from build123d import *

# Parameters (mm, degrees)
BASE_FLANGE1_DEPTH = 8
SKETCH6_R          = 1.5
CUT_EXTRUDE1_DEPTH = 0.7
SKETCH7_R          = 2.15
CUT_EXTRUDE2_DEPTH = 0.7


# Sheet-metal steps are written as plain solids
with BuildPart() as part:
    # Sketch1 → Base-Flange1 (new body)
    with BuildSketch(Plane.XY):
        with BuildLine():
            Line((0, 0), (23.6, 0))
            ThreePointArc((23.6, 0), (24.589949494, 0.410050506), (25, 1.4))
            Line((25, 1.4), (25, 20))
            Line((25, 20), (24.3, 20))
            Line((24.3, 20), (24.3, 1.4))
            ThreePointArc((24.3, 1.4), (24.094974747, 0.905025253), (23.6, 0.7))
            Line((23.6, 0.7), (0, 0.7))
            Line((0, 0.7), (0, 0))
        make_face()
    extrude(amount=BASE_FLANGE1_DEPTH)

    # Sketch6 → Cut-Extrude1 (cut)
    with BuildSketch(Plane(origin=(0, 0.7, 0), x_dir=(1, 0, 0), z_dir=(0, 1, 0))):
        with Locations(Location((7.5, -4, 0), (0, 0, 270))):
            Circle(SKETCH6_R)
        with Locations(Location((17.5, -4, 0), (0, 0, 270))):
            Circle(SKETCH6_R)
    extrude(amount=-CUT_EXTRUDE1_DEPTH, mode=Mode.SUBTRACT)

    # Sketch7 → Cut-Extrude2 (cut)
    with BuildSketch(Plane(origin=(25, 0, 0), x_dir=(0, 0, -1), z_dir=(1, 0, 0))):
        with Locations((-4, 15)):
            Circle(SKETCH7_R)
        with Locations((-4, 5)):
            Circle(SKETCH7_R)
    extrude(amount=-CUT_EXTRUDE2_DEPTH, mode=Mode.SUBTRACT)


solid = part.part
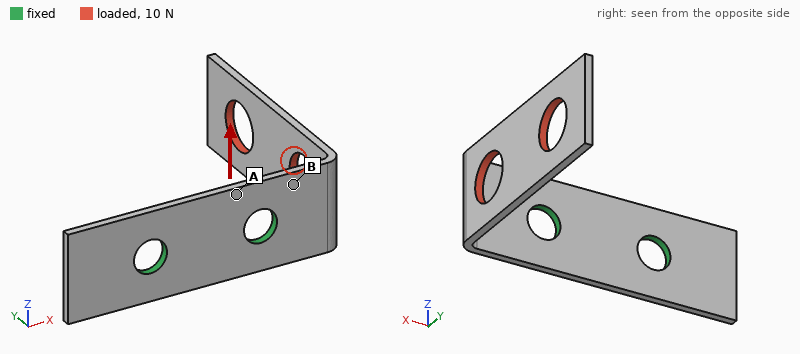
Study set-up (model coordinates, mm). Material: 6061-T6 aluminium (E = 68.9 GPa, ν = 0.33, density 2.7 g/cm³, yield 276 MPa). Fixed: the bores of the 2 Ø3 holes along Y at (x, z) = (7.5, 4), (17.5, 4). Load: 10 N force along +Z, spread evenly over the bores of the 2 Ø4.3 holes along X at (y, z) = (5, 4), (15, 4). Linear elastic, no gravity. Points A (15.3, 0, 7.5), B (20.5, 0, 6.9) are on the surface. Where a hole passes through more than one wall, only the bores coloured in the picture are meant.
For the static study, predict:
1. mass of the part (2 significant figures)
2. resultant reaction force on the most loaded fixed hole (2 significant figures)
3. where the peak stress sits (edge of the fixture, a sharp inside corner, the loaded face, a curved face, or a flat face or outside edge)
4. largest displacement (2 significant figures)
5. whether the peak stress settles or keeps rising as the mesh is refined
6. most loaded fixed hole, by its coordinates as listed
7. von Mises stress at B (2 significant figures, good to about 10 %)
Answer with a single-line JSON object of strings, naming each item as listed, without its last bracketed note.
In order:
{"mass of the part": "0.58 g", "resultant reaction force on the most loaded fixed hole": "12 N", "where the peak stress sits": "edge of the fixture", "largest displacement": "0.39 mm", "whether the peak stress settles or keeps rising as the mesh is refined": "keeps rising", "most loaded fixed hole, by its coordinates as listed": "(17.5, 4)", "von Mises stress at B": "81 MPa"}
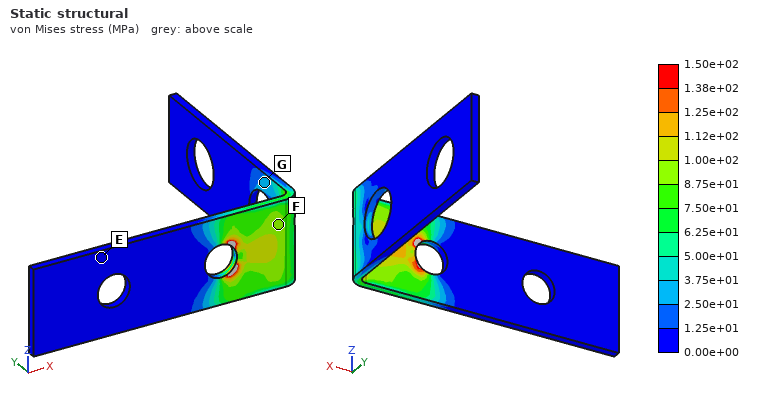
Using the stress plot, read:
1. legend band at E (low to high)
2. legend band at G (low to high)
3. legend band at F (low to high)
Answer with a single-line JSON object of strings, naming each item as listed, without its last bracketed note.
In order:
{"legend band at E": "0.00e+00 to 1.25e+01 MPa", "legend band at G": "2.50e+01 to 3.75e+01 MPa", "legend band at F": "8.75e+01 to 1.00e+02 MPa"}
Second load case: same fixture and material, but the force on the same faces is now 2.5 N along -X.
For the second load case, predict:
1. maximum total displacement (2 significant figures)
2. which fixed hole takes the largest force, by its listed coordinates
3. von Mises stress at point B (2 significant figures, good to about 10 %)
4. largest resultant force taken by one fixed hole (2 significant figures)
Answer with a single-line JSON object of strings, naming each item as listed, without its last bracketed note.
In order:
{"maximum total displacement": "0.36 mm", "which fixed hole takes the largest force, by its listed coordinates": "(17.5, 4)", "von Mises stress at point B": "33 MPa", "largest resultant force taken by one fixed hole": "2.4 N"}
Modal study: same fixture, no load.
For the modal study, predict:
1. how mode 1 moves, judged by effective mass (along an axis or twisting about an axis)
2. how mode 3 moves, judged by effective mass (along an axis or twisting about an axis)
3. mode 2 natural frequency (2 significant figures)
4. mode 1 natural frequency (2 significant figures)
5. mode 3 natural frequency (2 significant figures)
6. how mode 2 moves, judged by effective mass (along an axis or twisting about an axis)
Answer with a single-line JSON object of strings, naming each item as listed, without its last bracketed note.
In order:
{"how mode 1 moves, judged by effective mass": "along X", "how mode 3 moves, judged by effective mass": "along Y", "mode 2 natural frequency": "1900 Hz", "mode 1 natural frequency": "1000 Hz", "mode 3 natural frequency": "5100 Hz", "how mode 2 moves, judged by effective mass": "along Z"}
